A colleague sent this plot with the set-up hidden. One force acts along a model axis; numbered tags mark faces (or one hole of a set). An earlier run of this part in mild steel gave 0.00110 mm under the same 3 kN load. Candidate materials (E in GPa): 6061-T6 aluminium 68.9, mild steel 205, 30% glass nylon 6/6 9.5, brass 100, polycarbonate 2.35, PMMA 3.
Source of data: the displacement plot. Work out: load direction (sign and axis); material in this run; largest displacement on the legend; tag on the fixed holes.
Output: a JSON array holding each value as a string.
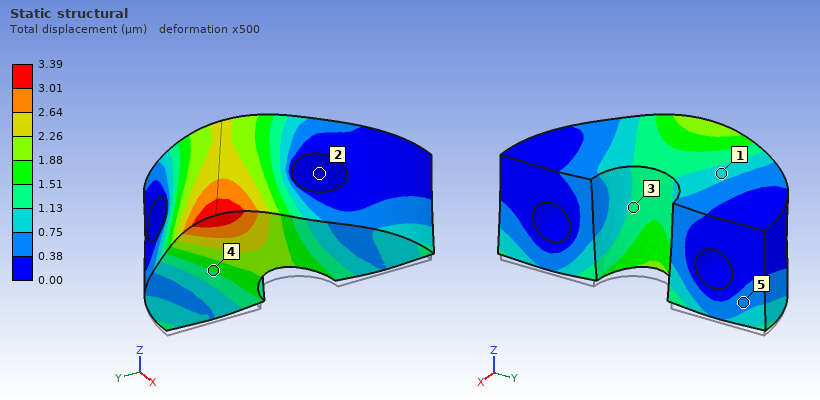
["+Z", "6061-T6 aluminium", "3.39 µm", "2"]
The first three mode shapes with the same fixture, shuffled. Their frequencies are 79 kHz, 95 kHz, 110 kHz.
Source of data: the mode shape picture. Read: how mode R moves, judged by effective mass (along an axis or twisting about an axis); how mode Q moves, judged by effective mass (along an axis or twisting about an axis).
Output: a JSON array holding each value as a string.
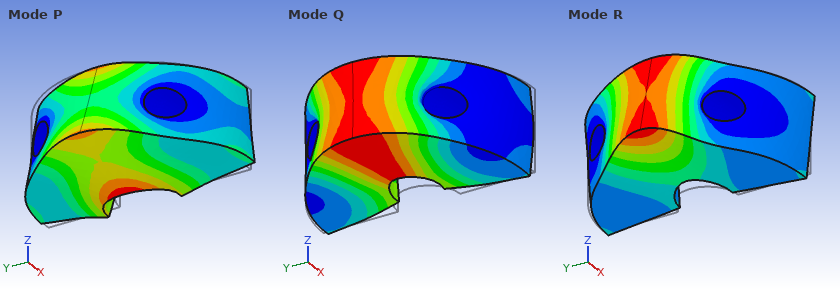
["along Z", "along X"]
